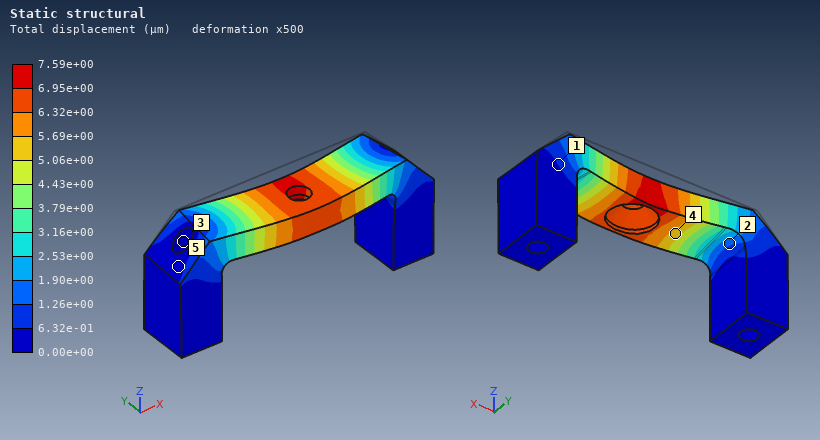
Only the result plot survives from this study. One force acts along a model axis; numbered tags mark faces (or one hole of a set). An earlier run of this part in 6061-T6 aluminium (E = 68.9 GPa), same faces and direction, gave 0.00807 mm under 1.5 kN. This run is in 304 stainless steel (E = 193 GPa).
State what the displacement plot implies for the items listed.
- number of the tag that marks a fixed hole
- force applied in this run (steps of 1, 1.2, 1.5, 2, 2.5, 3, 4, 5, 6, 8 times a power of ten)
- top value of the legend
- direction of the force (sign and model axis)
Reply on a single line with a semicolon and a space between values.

3; 4 kN; 7.59e+00 µm; -Y
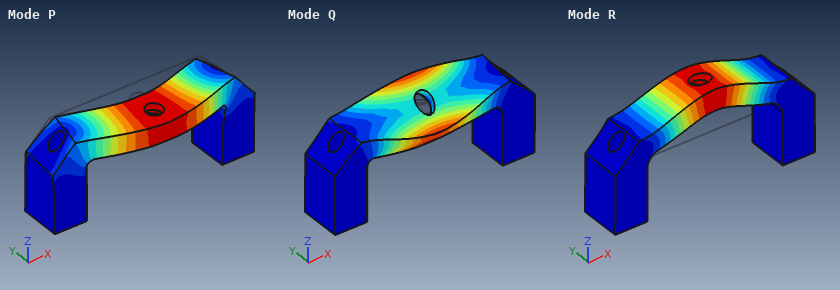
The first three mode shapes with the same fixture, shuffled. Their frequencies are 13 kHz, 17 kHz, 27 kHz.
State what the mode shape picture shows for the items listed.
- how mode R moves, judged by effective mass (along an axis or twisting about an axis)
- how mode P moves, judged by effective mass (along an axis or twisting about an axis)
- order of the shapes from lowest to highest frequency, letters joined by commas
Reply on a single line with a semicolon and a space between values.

along Z; along Y; R, P, Q
